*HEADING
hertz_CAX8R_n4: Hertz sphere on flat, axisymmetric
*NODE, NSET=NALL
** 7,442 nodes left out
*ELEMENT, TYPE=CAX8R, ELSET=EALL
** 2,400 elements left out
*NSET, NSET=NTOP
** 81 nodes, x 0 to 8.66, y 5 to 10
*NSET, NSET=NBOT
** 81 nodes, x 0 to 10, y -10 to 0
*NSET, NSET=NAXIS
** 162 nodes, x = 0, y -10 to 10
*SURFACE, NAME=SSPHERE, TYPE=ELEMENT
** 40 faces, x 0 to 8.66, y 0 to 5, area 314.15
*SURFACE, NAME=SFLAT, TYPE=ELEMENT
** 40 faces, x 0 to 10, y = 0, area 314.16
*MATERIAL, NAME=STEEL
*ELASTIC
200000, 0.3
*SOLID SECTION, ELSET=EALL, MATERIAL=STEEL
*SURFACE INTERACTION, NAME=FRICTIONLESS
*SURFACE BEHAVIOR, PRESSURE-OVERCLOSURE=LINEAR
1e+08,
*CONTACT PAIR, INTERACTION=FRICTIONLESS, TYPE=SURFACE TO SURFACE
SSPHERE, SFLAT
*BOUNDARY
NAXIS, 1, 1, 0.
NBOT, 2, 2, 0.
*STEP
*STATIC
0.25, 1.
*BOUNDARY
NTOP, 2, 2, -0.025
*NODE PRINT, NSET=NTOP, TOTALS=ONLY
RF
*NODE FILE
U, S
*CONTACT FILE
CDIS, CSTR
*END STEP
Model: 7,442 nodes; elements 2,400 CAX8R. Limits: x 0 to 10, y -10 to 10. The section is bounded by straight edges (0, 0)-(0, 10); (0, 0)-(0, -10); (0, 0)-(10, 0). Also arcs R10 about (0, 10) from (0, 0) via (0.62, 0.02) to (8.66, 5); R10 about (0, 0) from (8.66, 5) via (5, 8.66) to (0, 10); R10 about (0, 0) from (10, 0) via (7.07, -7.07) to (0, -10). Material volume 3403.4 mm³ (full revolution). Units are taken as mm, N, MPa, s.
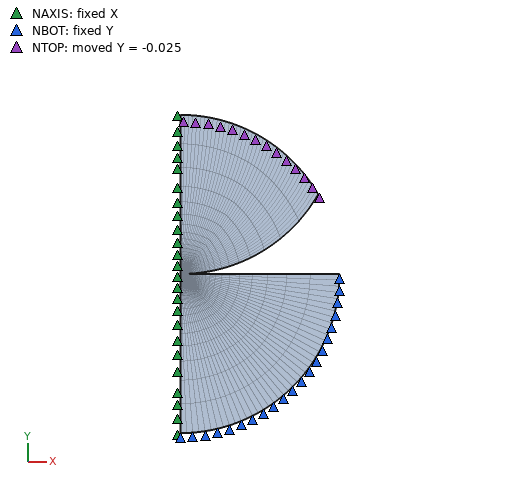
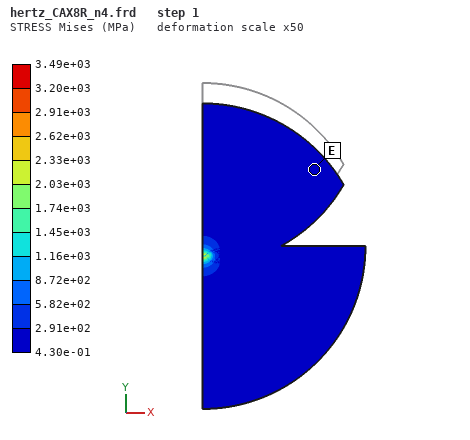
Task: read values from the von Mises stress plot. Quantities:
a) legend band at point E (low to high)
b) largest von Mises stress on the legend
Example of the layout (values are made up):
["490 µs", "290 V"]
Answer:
["4.30e-01 to 2.91e+02 MPa", "3.49e+03 MPa"]
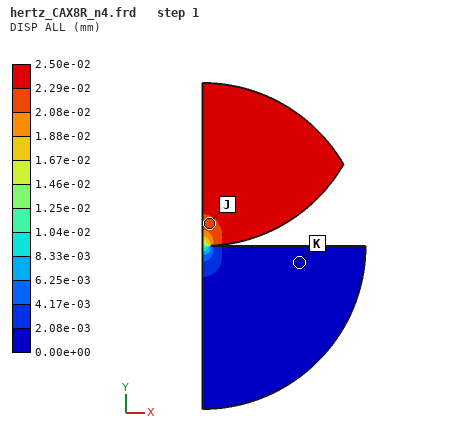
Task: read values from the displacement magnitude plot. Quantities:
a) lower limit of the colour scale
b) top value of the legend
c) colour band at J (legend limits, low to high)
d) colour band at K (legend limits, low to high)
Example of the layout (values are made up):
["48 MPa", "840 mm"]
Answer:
["0.00e+00 mm", "2.50e-02 mm", "2.08e-02 to 2.29e-02 mm", "0.00e+00 to 2.08e-03 mm"]
